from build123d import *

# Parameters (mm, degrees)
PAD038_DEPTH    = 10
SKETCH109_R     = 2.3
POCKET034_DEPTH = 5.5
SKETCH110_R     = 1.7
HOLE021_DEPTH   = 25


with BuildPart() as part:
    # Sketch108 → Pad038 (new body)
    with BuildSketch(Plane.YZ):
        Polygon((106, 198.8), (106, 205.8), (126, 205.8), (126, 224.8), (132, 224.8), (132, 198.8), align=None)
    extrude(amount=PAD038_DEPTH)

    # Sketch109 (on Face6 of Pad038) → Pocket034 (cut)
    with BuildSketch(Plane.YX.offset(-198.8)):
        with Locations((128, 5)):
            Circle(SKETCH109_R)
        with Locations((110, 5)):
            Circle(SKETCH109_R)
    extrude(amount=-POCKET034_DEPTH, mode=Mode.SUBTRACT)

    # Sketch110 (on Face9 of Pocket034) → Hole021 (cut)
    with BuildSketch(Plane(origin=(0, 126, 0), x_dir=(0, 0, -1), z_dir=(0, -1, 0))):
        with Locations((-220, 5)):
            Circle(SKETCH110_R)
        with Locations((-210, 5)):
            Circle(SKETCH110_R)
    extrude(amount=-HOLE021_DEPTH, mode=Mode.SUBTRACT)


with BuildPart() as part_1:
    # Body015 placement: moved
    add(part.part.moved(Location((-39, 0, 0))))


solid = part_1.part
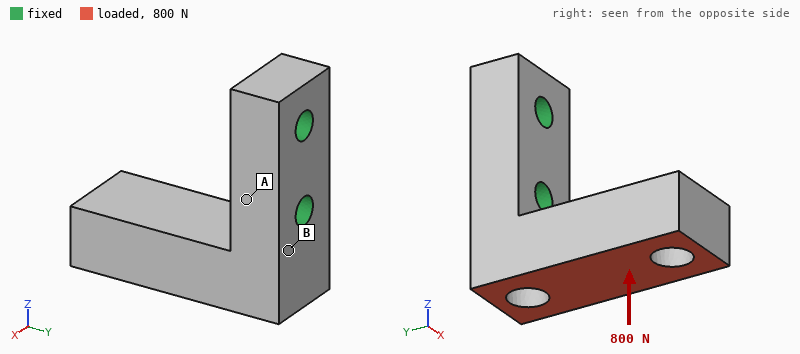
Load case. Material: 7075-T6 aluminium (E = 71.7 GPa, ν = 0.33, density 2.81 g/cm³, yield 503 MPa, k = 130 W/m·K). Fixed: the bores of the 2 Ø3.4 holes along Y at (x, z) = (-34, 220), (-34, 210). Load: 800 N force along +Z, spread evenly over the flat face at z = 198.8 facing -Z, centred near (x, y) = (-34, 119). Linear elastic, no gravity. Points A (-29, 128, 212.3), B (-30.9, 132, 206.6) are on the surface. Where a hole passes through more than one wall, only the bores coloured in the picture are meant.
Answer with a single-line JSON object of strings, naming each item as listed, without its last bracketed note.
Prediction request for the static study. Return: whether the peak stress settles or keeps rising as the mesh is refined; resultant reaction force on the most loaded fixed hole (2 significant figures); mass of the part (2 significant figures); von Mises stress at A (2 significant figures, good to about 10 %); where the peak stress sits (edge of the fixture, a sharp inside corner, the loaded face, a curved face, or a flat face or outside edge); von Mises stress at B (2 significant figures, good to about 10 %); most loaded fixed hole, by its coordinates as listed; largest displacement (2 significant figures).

{"whether the peak stress settles or keeps rising as the mesh is refined": "keeps rising", "resultant reaction force on the most loaded fixed hole": "720 N", "mass of the part": "7.5 g", "von Mises stress at A": "28 MPa", "where the peak stress sits": "edge of the fixture", "von Mises stress at B": "110 MPa", "most loaded fixed hole, by its coordinates as listed": "(-34, 210)", "largest displacement": "0.16 mm"}
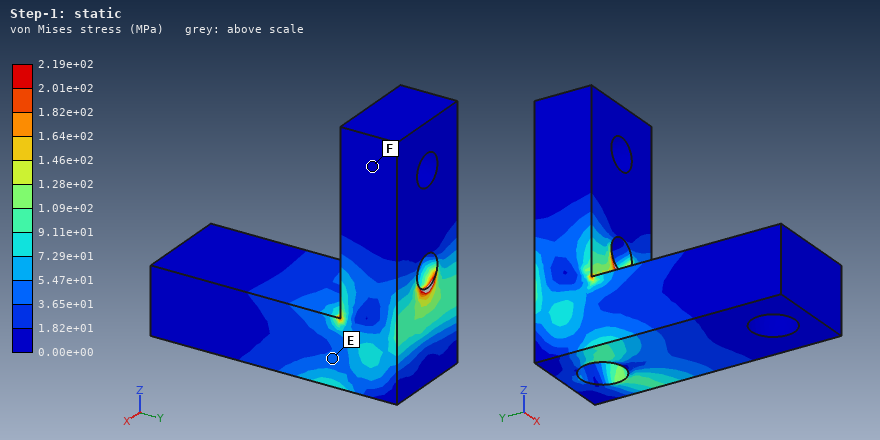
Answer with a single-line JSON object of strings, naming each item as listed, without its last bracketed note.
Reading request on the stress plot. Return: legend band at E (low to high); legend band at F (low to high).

{"legend band at E": "3.65e+01 to 5.47e+01 MPa", "legend band at F": "0.00e+00 to 1.82e+01 MPa"}
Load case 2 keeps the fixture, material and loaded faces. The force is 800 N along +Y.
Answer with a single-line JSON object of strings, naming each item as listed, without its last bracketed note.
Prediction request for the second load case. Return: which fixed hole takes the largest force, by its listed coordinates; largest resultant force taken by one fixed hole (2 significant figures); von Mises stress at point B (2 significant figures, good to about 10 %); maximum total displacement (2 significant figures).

{"which fixed hole takes the largest force, by its listed coordinates": "(-34, 210)", "largest resultant force taken by one fixed hole": "920 N", "von Mises stress at point B": "90 MPa", "maximum total displacement": "0.11 mm"}
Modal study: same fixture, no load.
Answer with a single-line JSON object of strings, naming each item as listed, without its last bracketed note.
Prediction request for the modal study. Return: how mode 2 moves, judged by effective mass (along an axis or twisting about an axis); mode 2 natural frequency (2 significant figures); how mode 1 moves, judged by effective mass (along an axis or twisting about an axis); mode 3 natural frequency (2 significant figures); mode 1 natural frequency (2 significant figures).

{"how mode 2 moves, judged by effective mass": "along X", "mode 2 natural frequency": "7700 Hz", "how mode 1 moves, judged by effective mass": "along Z", "mode 3 natural frequency": "22 kHz", "mode 1 natural frequency": "6400 Hz"}
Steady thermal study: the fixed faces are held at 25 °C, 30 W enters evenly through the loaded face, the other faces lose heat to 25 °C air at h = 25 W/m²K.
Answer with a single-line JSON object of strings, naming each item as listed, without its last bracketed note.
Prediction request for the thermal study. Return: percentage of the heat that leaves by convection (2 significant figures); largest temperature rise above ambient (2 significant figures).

{"percentage of the heat that leaves by convection": "3.2 %", "largest temperature rise above ambient": "58 K"}
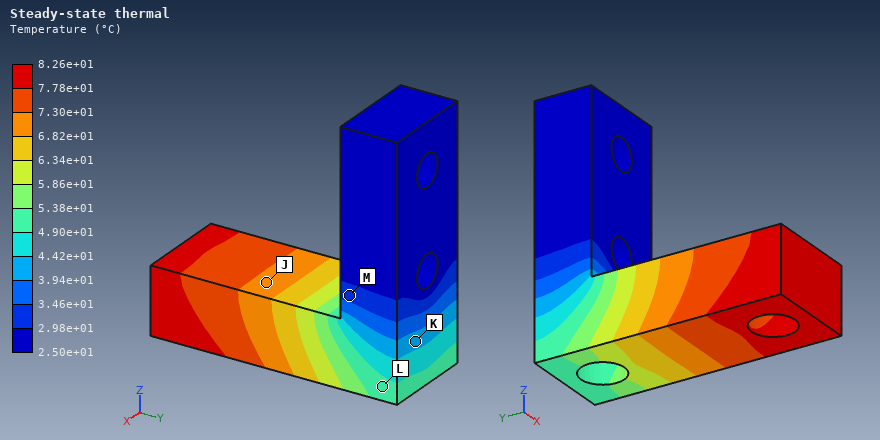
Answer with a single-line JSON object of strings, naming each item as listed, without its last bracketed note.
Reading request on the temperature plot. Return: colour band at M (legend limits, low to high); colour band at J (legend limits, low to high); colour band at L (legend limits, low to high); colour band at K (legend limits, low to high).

{"colour band at M": "2.98e+01 to 3.46e+01 °C", "colour band at J": "6.82e+01 to 7.30e+01 °C", "colour band at L": "4.90e+01 to 5.38e+01 °C", "colour band at K": "3.94e+01 to 4.42e+01 °C"}
